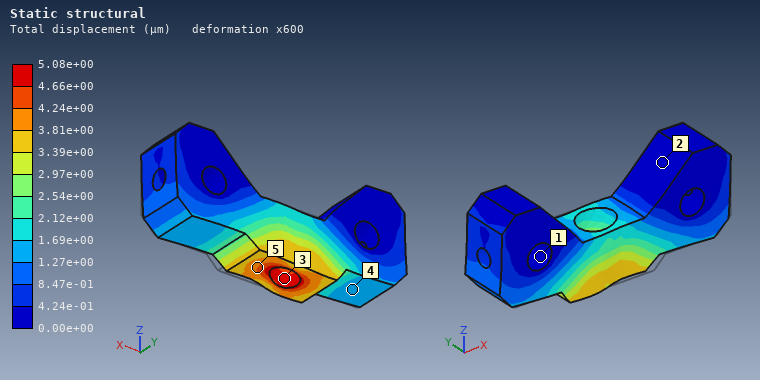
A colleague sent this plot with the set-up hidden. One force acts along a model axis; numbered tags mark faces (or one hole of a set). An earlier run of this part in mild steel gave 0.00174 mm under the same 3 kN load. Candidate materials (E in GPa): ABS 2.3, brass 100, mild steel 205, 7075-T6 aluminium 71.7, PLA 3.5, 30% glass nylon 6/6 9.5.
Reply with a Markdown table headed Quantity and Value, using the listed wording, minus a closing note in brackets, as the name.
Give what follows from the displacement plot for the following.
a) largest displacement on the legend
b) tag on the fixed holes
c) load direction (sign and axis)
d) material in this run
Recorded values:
| Quantity | Value |
|---|---|
| largest displacement on the legend | 5.08e+00 µm |
| tag on the fixed holes | 1 |
| load direction | -X |
| material in this run | 7075-T6 aluminium |
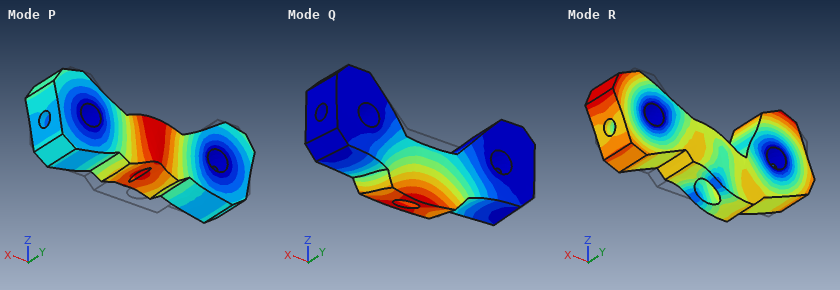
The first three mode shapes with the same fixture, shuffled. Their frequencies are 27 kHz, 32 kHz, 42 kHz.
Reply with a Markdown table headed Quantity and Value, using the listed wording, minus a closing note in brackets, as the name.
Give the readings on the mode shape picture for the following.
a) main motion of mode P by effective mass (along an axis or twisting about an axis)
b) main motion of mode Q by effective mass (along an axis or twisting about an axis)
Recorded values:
| Quantity | Value |
|---|---|
| main motion of mode P by effective mass | along Z |
| main motion of mode Q by effective mass | along Y |
